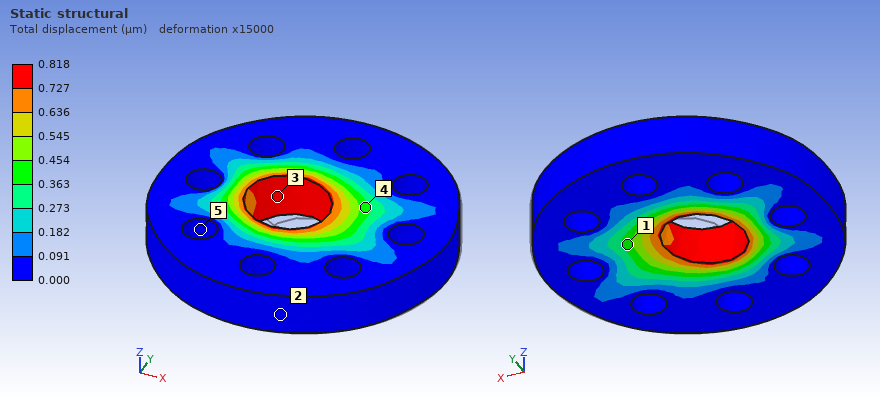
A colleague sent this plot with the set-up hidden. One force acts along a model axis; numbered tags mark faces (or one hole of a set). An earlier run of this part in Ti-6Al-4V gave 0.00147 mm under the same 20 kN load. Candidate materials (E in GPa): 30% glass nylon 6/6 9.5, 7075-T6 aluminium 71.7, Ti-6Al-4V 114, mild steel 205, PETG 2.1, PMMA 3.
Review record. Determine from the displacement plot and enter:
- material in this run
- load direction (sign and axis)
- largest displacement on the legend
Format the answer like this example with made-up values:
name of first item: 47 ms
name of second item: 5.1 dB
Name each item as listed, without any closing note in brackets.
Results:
material in this run: mild steel
load direction: -X
largest displacement on the legend: 0.818 µm
